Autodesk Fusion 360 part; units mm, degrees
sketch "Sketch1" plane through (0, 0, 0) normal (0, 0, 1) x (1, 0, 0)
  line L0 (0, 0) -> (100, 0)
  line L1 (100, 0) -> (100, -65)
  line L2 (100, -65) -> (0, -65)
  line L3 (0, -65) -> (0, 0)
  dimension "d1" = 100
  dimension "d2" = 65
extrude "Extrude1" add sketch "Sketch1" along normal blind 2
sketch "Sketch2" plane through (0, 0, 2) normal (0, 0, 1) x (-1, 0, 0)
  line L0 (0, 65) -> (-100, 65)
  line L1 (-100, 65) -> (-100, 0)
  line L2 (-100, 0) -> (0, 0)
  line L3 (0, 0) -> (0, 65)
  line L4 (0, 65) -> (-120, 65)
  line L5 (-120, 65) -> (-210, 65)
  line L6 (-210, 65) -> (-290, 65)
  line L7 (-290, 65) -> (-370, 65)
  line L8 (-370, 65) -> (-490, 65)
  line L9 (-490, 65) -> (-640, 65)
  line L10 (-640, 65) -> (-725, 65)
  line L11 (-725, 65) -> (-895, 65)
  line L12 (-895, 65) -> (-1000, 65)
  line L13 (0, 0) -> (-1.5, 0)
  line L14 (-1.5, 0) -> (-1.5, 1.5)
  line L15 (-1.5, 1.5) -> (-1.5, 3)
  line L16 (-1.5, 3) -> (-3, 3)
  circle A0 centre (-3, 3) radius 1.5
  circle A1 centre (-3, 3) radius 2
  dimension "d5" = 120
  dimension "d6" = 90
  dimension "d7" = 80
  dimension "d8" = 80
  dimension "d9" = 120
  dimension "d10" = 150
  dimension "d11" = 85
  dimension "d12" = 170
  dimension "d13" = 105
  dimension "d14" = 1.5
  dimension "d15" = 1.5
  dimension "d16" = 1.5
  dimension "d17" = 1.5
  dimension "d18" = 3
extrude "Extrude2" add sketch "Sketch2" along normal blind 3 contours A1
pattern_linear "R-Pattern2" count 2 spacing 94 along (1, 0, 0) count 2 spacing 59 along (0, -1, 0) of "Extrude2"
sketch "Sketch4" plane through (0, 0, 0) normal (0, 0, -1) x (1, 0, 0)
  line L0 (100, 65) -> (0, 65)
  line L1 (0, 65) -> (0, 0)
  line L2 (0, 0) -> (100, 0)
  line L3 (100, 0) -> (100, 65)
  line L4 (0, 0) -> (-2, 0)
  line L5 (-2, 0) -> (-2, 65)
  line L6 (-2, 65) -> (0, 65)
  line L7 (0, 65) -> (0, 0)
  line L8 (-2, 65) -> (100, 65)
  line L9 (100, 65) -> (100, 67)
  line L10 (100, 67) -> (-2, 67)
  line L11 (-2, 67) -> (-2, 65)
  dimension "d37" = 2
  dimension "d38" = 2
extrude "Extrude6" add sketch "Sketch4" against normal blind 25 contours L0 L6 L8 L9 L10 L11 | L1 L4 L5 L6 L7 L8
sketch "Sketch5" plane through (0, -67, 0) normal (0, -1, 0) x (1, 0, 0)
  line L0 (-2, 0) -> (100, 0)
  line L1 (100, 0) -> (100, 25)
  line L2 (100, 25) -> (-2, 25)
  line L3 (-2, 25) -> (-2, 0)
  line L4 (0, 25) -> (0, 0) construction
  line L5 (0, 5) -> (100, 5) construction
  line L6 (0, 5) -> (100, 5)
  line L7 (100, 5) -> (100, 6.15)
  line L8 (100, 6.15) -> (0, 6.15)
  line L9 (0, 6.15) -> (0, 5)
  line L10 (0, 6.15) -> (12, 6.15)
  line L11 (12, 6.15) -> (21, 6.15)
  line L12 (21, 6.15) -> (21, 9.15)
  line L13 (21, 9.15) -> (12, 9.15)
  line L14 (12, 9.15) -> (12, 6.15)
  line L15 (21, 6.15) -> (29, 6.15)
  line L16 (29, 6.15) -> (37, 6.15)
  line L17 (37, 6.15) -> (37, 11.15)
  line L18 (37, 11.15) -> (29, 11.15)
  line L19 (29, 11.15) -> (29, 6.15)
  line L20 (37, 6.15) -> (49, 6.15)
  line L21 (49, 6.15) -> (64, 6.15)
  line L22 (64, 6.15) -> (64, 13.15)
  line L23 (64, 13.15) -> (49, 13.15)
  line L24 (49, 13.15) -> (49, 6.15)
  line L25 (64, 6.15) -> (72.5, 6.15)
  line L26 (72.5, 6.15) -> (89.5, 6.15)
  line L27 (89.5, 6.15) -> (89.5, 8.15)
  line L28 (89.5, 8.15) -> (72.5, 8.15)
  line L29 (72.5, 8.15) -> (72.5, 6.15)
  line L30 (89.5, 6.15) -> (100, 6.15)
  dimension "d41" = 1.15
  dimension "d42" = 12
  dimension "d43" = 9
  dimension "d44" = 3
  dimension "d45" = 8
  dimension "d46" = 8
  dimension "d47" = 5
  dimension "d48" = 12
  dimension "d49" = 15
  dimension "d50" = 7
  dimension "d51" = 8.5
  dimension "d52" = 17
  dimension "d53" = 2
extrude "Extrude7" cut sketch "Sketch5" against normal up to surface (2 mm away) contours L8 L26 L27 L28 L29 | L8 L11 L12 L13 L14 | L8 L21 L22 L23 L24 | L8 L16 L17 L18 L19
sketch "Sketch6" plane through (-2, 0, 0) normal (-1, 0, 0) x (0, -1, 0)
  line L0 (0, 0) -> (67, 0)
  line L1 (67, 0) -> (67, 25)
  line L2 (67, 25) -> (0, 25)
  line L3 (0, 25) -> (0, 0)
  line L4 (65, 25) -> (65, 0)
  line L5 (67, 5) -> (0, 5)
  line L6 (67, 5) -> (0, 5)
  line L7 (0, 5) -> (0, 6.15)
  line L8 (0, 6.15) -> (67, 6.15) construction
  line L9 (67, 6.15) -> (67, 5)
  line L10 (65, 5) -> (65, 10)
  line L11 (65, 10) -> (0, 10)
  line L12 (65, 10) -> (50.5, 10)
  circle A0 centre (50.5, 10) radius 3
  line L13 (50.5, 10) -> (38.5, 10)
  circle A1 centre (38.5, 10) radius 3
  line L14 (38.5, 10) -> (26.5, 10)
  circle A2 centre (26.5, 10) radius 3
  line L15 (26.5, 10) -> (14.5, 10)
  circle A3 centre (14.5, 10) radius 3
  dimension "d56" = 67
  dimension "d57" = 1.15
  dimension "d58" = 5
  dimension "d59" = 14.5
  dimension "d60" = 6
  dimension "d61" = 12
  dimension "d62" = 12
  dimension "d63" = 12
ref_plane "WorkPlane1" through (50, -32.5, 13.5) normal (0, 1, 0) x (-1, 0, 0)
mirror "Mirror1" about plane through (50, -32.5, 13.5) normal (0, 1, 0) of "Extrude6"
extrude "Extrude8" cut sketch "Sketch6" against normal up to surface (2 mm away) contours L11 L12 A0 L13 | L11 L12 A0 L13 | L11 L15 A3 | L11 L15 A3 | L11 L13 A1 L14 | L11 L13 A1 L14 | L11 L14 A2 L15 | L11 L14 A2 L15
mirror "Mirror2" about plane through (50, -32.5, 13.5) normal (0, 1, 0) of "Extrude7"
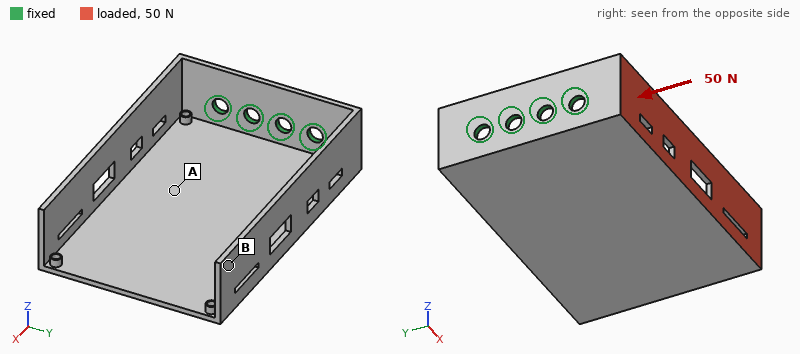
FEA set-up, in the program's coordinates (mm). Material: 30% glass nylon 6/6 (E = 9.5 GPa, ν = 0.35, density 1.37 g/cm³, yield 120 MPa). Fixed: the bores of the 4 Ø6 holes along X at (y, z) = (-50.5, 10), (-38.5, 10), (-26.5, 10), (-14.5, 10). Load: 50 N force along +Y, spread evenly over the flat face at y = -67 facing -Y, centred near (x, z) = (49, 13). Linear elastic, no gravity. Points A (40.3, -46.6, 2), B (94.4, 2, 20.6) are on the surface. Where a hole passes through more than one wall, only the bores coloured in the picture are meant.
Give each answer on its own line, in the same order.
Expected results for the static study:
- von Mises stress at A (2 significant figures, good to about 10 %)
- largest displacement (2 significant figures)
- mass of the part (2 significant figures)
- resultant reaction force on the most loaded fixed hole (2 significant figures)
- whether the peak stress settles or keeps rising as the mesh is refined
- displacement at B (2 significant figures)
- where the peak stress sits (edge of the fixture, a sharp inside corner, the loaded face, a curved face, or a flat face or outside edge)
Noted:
4.2 MPa
1.4 mm
35 g
60 N
keeps rising
0.81 mm
edge of the fixture
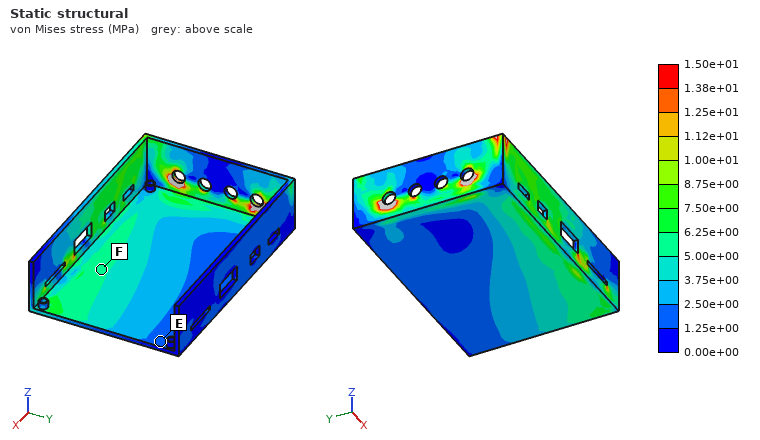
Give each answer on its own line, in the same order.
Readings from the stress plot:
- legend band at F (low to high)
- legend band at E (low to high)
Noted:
5.00e+00 to 6.25e+00 MPa
1.25e+00 to 2.50e+00 MPa
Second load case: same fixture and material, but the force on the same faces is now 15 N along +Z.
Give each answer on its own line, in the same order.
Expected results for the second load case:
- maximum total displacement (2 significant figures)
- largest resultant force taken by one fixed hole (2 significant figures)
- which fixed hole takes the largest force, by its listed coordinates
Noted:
1.2 mm
25 N
(-50.5, 10)
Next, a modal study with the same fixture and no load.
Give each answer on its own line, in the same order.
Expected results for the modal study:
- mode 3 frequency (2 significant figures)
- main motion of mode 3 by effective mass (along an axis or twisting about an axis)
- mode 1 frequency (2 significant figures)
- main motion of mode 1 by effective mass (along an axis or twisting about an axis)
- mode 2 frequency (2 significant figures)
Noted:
580 Hz
along Y
150 Hz
along Z
230 Hz
